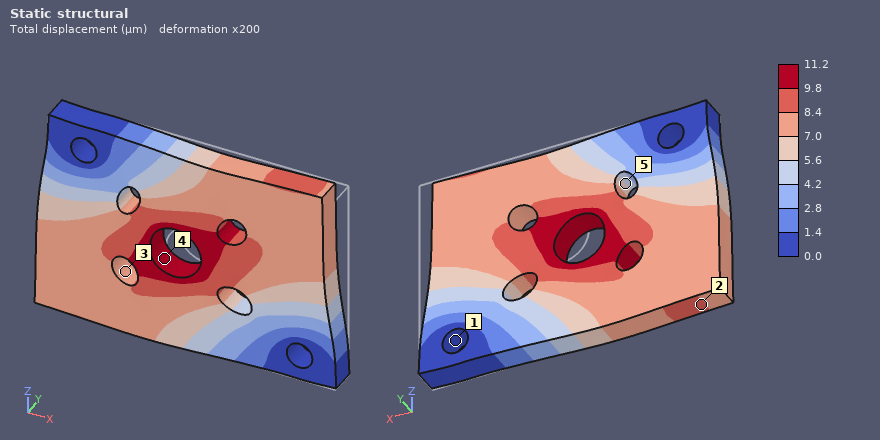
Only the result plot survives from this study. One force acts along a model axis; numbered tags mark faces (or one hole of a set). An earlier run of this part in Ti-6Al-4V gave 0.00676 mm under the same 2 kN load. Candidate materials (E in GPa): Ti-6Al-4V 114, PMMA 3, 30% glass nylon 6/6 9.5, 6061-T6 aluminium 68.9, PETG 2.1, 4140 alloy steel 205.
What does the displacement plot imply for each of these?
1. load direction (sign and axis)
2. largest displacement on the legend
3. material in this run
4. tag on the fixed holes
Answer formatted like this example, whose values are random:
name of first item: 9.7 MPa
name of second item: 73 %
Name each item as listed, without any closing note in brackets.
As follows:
load direction: -X
largest displacement on the legend: 11.2 µm
material in this run: 6061-T6 aluminium
tag on the fixed holes: 1
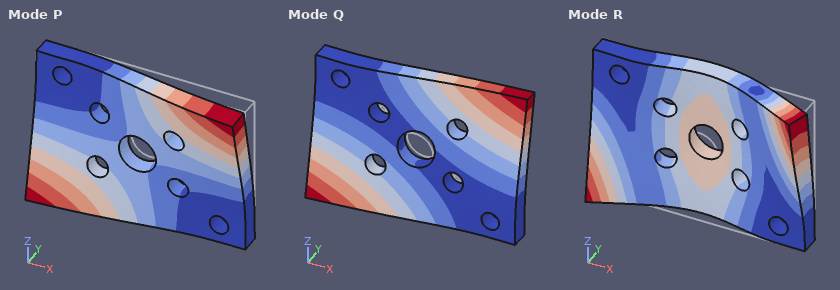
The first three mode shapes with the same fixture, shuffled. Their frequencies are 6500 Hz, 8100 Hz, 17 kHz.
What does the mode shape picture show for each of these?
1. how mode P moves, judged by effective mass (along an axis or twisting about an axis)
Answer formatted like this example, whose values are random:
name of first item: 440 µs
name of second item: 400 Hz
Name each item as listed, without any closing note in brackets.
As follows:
how mode P moves, judged by effective mass: along Y
